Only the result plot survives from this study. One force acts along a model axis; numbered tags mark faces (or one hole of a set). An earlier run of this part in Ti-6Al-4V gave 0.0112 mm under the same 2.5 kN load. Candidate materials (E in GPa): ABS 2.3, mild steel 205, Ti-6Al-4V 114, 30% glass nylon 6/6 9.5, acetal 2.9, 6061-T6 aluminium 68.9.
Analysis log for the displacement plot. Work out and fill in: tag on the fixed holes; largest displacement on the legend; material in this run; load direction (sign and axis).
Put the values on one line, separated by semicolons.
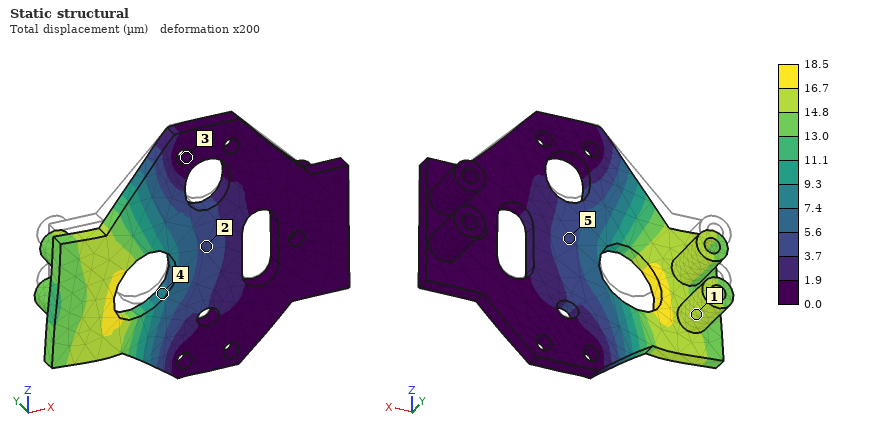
3; 18.5 µm; 6061-T6 aluminium; -Z
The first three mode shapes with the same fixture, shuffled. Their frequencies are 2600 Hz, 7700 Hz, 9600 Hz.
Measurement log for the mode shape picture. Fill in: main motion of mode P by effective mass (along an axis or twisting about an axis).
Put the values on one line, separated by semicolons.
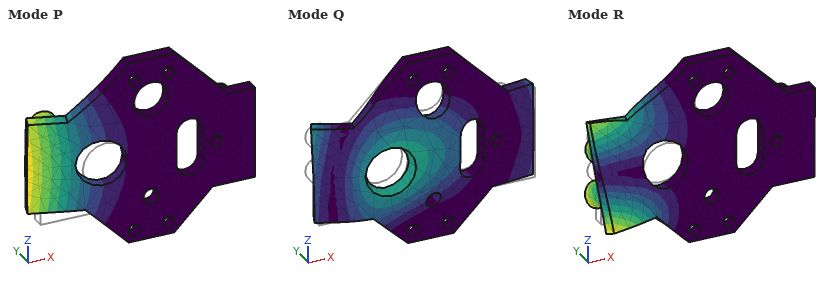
along Y
